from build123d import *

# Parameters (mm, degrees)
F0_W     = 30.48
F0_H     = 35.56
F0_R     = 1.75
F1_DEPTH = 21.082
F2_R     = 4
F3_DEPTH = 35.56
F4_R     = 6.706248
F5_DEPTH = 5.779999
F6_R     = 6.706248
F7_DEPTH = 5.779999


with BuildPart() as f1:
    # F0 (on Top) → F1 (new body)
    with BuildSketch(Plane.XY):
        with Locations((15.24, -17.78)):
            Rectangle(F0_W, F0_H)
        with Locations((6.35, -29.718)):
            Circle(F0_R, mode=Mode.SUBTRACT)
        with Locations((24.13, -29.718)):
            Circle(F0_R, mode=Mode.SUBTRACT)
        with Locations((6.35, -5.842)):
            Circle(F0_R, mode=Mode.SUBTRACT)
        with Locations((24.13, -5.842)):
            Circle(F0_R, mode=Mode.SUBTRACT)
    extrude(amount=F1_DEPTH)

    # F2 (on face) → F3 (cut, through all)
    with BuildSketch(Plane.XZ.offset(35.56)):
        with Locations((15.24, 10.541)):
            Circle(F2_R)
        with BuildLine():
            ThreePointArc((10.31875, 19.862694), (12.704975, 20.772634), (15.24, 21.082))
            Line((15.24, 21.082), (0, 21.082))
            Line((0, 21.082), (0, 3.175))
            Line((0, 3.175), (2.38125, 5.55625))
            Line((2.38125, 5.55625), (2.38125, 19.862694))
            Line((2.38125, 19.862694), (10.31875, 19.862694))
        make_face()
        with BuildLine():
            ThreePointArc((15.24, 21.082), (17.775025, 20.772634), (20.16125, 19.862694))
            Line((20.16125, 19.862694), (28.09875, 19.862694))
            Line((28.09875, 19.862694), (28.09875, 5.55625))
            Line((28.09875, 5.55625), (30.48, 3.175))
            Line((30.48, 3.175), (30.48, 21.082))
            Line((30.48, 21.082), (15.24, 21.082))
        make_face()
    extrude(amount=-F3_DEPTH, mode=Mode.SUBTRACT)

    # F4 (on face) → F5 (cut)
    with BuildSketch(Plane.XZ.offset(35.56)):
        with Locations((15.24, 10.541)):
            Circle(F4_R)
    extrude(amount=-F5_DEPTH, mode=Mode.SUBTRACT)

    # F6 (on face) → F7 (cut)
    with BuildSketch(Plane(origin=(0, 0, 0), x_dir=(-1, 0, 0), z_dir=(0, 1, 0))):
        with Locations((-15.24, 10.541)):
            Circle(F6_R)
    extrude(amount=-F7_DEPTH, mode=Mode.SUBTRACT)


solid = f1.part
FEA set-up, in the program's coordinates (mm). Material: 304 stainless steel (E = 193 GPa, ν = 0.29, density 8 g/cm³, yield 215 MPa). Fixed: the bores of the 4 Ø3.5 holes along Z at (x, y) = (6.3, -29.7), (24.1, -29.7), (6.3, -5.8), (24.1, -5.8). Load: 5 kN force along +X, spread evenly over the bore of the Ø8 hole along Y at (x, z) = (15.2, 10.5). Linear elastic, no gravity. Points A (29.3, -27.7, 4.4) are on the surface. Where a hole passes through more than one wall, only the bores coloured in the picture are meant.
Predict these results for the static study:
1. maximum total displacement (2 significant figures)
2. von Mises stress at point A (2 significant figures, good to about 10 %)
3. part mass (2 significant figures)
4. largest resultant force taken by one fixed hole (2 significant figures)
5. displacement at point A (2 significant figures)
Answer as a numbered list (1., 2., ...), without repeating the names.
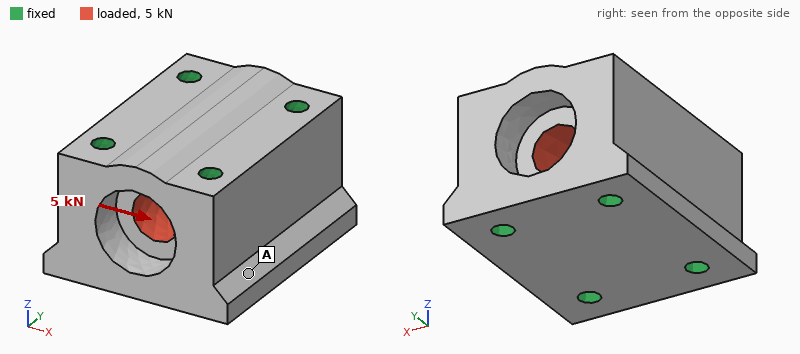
1. 0.74 µm
2. 3.2 MPa
3. 120 g
4. 1.3 kN
5. 0.16 µm
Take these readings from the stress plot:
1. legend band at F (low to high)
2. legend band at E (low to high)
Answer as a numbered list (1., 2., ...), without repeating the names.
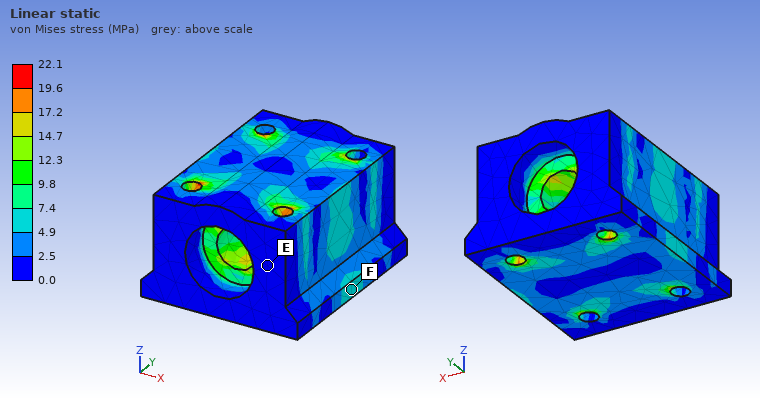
1. 4.9 to 7.4 MPa
2. 0.0 to 2.5 MPa
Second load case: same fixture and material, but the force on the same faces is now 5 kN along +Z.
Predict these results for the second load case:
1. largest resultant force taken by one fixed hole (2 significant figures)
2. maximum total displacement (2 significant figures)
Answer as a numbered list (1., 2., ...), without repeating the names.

1. 1.3 kN
2. 1.0 µm
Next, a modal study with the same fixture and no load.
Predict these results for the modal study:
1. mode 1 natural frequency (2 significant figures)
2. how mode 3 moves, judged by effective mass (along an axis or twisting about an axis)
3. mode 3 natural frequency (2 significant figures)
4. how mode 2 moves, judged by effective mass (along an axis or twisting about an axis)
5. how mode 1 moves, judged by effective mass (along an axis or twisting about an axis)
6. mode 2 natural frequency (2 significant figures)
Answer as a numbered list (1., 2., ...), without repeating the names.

1. 53 kHz
2. twisting about Y
3. 60 kHz
4. along X
5. along Z
6. 56 kHz
